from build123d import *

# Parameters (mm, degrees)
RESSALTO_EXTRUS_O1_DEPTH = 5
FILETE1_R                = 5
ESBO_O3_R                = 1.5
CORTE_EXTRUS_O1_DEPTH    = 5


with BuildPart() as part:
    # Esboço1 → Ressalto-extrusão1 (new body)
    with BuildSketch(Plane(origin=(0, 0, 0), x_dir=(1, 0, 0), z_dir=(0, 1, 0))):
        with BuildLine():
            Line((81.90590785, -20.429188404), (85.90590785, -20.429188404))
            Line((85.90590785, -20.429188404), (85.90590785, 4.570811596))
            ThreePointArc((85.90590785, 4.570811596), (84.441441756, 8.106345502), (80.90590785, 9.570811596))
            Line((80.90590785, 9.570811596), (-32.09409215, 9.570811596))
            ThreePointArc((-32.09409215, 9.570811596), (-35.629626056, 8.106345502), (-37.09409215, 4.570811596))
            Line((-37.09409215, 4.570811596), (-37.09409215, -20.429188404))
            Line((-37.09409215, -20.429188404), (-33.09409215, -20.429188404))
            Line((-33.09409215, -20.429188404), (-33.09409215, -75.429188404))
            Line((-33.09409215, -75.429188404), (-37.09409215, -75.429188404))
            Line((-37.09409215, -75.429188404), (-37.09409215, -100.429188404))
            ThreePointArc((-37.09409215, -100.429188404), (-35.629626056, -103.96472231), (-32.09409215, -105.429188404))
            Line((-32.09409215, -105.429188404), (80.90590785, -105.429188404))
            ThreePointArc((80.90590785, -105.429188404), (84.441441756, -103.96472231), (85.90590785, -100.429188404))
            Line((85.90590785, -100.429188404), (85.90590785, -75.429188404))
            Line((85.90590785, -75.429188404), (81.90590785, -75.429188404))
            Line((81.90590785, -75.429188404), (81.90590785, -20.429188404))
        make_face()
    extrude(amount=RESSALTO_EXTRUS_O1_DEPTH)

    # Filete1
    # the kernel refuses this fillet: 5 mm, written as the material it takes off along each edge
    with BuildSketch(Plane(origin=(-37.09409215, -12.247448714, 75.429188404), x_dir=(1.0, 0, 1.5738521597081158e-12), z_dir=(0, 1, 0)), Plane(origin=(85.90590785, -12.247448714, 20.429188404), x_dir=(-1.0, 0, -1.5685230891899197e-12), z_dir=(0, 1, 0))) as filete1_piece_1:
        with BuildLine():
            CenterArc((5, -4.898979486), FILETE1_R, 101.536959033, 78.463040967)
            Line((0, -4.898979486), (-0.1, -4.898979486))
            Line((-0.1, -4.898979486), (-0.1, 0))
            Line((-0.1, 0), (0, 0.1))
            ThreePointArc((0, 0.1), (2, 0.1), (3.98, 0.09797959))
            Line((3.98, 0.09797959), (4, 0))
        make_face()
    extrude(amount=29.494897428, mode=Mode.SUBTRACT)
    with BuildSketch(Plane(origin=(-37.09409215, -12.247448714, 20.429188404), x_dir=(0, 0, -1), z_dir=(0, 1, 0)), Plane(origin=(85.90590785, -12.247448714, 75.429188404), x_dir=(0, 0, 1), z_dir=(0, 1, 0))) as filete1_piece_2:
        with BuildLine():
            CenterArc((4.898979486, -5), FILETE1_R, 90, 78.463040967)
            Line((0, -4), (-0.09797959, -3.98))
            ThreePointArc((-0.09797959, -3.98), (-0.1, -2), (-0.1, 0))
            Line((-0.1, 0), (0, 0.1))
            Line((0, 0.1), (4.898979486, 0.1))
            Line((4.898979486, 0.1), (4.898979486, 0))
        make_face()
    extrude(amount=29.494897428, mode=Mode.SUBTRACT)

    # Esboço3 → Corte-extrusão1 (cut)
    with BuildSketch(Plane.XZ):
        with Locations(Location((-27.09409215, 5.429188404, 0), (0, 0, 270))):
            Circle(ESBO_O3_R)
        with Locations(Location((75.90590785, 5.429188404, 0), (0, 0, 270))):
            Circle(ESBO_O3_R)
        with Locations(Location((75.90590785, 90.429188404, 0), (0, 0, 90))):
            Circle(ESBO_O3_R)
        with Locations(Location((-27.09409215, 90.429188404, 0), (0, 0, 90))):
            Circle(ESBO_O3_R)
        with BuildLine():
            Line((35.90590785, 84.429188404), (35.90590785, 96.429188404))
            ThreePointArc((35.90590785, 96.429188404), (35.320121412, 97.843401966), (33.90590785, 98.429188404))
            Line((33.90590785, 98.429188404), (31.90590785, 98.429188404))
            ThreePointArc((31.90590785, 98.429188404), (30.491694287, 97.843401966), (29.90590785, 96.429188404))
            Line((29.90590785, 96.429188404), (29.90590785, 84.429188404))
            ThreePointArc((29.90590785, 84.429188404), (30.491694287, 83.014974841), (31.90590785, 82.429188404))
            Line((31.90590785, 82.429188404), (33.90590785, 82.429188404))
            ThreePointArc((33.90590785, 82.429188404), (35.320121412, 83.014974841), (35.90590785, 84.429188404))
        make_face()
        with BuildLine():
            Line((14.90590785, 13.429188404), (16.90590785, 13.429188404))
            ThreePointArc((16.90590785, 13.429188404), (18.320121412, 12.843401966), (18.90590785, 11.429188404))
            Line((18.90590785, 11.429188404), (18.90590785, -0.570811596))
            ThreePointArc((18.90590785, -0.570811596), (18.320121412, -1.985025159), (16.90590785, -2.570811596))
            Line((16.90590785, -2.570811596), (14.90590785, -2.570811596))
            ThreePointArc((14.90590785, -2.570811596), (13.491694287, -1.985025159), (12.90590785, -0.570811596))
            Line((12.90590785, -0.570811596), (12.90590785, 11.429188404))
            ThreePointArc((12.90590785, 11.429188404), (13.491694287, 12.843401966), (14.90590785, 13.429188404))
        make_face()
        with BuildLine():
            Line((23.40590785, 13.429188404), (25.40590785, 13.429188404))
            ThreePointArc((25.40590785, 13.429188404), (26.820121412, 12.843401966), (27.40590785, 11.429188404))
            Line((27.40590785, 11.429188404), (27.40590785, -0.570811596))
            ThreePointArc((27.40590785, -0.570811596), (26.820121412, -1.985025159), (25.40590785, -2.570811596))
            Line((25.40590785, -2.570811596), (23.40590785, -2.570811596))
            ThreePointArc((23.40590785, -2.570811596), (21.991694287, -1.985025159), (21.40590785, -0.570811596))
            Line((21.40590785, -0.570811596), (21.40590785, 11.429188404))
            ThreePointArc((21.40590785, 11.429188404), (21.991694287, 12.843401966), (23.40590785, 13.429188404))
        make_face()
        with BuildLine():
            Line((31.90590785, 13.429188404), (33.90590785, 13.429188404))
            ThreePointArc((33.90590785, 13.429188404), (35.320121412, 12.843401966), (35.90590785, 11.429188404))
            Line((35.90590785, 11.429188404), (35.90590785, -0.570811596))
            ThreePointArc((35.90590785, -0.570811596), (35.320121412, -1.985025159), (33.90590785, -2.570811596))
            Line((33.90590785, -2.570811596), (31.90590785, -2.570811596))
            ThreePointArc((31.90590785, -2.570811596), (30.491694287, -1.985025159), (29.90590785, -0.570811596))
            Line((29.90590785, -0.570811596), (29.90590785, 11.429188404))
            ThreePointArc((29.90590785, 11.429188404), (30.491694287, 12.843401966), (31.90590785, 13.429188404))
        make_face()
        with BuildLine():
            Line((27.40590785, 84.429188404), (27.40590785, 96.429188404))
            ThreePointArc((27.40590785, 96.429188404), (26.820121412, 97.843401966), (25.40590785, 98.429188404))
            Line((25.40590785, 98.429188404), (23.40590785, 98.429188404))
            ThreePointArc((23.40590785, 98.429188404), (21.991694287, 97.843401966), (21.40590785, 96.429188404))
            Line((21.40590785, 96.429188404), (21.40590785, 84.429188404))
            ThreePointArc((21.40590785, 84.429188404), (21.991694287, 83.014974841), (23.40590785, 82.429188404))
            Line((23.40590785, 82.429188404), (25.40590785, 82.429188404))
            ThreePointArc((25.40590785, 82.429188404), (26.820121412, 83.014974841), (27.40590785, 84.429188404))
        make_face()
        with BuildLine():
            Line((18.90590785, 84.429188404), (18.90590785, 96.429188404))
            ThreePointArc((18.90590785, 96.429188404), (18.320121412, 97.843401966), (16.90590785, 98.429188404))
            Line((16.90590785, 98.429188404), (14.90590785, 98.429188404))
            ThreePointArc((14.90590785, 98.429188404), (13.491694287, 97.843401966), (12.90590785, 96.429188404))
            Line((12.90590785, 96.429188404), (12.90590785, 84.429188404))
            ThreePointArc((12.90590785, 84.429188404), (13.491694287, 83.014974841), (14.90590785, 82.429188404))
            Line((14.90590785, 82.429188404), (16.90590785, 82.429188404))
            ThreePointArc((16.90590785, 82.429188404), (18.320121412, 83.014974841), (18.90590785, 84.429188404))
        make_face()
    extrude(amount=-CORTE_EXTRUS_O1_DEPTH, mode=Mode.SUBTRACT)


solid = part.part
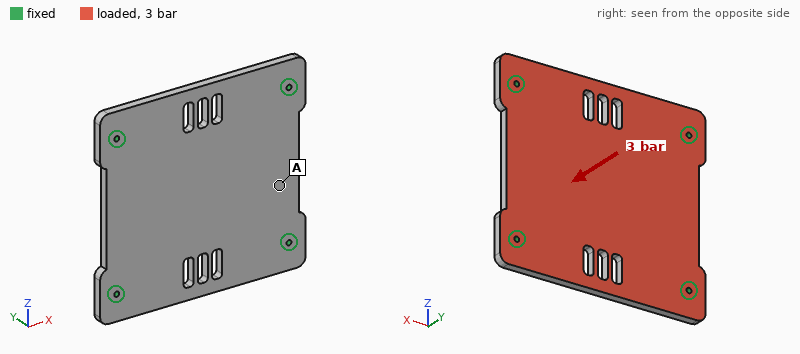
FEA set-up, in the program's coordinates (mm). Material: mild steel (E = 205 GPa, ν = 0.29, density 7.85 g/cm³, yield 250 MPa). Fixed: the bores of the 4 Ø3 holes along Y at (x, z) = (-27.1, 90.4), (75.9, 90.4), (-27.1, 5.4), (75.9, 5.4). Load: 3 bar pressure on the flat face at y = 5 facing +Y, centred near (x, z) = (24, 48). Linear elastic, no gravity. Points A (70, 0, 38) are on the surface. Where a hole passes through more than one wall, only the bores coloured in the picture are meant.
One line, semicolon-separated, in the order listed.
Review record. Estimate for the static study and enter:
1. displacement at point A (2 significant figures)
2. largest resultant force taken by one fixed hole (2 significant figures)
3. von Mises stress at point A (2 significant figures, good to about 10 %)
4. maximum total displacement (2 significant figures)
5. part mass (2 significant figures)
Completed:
40 µm; 980 N; 28 MPa; 97 µm; 510 g
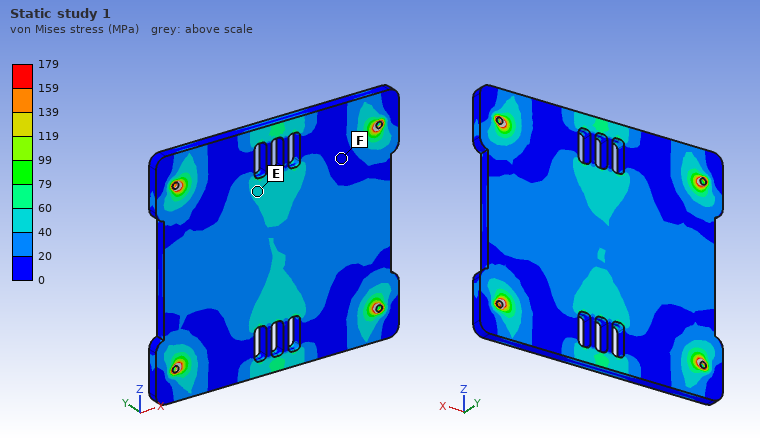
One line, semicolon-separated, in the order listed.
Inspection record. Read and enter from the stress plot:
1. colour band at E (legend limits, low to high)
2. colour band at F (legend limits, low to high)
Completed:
40 to 60 MPa; 0 to 20 MPa
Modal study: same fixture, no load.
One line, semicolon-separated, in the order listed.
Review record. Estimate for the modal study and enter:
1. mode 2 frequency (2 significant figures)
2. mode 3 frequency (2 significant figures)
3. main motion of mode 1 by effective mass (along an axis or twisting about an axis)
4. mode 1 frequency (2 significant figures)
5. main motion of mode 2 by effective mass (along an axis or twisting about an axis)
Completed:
2600 Hz; 3200 Hz; along Y; 1700 Hz; twisting about X
